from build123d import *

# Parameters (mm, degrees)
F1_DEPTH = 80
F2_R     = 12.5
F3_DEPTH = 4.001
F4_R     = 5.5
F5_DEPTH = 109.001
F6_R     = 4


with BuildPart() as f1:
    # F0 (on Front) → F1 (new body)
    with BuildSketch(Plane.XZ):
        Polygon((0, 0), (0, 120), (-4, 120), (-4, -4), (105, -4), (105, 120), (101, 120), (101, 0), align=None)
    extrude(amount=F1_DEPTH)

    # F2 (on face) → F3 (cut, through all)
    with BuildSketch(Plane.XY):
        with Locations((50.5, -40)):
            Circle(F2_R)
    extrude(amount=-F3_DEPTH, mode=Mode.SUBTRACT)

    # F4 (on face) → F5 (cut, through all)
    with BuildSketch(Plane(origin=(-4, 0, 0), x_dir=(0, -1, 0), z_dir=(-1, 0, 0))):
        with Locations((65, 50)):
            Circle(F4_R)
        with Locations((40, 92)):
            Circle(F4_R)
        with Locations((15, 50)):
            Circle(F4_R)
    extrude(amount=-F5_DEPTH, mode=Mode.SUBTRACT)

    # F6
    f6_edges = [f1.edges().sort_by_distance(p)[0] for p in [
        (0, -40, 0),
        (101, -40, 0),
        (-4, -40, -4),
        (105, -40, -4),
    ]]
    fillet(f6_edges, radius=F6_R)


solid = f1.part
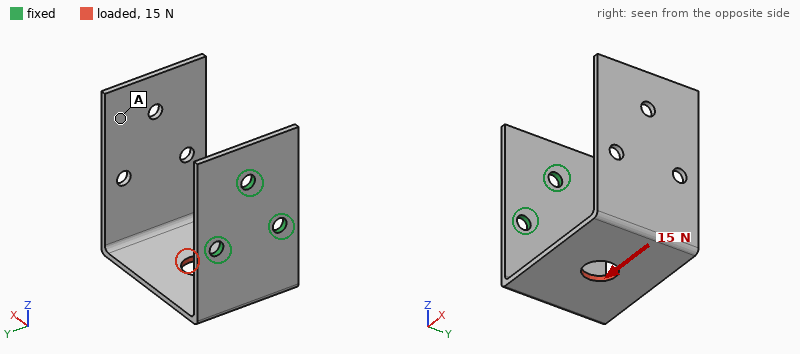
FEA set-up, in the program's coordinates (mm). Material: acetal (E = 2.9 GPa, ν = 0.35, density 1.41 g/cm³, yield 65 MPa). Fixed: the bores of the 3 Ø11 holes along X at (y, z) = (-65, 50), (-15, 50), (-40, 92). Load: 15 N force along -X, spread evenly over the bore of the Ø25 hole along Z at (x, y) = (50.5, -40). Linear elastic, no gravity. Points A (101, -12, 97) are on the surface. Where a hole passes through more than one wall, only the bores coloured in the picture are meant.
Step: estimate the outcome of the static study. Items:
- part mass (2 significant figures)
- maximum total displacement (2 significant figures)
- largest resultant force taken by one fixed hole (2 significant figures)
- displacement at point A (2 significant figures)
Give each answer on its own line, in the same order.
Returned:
150 g
1.9 mm
8.4 N
1.7 mm
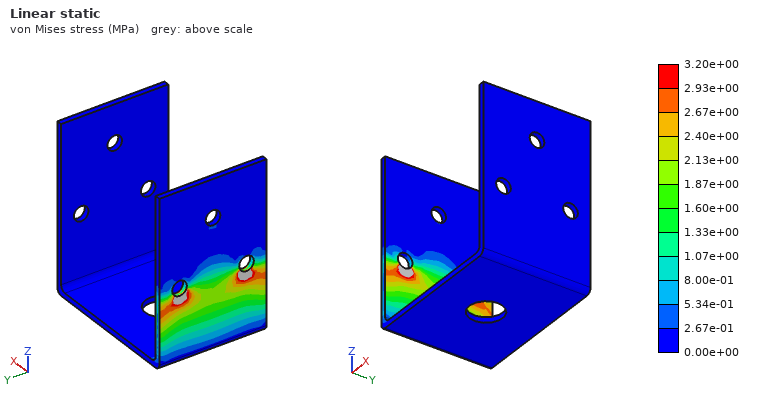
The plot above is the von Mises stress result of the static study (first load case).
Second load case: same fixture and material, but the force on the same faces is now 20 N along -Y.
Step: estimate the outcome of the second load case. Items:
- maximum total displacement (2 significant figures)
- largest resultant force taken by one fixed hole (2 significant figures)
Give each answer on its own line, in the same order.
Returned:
2.0 mm
27 N
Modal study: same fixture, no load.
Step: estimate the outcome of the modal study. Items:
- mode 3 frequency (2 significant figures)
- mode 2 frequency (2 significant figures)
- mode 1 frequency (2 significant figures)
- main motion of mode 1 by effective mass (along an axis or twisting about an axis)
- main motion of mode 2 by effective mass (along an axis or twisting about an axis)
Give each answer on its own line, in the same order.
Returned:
50 Hz
32 Hz
19 Hz
along Z
along Y
